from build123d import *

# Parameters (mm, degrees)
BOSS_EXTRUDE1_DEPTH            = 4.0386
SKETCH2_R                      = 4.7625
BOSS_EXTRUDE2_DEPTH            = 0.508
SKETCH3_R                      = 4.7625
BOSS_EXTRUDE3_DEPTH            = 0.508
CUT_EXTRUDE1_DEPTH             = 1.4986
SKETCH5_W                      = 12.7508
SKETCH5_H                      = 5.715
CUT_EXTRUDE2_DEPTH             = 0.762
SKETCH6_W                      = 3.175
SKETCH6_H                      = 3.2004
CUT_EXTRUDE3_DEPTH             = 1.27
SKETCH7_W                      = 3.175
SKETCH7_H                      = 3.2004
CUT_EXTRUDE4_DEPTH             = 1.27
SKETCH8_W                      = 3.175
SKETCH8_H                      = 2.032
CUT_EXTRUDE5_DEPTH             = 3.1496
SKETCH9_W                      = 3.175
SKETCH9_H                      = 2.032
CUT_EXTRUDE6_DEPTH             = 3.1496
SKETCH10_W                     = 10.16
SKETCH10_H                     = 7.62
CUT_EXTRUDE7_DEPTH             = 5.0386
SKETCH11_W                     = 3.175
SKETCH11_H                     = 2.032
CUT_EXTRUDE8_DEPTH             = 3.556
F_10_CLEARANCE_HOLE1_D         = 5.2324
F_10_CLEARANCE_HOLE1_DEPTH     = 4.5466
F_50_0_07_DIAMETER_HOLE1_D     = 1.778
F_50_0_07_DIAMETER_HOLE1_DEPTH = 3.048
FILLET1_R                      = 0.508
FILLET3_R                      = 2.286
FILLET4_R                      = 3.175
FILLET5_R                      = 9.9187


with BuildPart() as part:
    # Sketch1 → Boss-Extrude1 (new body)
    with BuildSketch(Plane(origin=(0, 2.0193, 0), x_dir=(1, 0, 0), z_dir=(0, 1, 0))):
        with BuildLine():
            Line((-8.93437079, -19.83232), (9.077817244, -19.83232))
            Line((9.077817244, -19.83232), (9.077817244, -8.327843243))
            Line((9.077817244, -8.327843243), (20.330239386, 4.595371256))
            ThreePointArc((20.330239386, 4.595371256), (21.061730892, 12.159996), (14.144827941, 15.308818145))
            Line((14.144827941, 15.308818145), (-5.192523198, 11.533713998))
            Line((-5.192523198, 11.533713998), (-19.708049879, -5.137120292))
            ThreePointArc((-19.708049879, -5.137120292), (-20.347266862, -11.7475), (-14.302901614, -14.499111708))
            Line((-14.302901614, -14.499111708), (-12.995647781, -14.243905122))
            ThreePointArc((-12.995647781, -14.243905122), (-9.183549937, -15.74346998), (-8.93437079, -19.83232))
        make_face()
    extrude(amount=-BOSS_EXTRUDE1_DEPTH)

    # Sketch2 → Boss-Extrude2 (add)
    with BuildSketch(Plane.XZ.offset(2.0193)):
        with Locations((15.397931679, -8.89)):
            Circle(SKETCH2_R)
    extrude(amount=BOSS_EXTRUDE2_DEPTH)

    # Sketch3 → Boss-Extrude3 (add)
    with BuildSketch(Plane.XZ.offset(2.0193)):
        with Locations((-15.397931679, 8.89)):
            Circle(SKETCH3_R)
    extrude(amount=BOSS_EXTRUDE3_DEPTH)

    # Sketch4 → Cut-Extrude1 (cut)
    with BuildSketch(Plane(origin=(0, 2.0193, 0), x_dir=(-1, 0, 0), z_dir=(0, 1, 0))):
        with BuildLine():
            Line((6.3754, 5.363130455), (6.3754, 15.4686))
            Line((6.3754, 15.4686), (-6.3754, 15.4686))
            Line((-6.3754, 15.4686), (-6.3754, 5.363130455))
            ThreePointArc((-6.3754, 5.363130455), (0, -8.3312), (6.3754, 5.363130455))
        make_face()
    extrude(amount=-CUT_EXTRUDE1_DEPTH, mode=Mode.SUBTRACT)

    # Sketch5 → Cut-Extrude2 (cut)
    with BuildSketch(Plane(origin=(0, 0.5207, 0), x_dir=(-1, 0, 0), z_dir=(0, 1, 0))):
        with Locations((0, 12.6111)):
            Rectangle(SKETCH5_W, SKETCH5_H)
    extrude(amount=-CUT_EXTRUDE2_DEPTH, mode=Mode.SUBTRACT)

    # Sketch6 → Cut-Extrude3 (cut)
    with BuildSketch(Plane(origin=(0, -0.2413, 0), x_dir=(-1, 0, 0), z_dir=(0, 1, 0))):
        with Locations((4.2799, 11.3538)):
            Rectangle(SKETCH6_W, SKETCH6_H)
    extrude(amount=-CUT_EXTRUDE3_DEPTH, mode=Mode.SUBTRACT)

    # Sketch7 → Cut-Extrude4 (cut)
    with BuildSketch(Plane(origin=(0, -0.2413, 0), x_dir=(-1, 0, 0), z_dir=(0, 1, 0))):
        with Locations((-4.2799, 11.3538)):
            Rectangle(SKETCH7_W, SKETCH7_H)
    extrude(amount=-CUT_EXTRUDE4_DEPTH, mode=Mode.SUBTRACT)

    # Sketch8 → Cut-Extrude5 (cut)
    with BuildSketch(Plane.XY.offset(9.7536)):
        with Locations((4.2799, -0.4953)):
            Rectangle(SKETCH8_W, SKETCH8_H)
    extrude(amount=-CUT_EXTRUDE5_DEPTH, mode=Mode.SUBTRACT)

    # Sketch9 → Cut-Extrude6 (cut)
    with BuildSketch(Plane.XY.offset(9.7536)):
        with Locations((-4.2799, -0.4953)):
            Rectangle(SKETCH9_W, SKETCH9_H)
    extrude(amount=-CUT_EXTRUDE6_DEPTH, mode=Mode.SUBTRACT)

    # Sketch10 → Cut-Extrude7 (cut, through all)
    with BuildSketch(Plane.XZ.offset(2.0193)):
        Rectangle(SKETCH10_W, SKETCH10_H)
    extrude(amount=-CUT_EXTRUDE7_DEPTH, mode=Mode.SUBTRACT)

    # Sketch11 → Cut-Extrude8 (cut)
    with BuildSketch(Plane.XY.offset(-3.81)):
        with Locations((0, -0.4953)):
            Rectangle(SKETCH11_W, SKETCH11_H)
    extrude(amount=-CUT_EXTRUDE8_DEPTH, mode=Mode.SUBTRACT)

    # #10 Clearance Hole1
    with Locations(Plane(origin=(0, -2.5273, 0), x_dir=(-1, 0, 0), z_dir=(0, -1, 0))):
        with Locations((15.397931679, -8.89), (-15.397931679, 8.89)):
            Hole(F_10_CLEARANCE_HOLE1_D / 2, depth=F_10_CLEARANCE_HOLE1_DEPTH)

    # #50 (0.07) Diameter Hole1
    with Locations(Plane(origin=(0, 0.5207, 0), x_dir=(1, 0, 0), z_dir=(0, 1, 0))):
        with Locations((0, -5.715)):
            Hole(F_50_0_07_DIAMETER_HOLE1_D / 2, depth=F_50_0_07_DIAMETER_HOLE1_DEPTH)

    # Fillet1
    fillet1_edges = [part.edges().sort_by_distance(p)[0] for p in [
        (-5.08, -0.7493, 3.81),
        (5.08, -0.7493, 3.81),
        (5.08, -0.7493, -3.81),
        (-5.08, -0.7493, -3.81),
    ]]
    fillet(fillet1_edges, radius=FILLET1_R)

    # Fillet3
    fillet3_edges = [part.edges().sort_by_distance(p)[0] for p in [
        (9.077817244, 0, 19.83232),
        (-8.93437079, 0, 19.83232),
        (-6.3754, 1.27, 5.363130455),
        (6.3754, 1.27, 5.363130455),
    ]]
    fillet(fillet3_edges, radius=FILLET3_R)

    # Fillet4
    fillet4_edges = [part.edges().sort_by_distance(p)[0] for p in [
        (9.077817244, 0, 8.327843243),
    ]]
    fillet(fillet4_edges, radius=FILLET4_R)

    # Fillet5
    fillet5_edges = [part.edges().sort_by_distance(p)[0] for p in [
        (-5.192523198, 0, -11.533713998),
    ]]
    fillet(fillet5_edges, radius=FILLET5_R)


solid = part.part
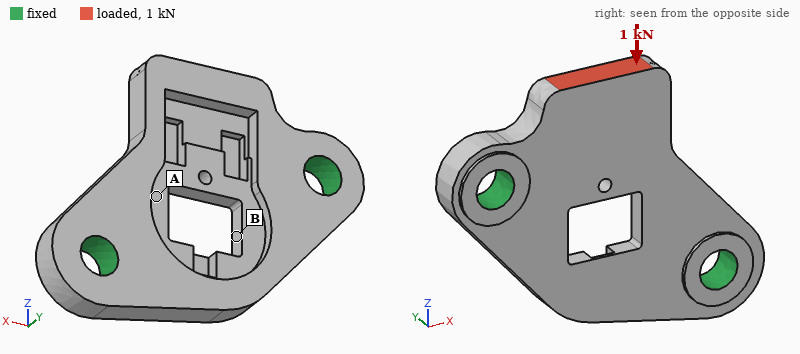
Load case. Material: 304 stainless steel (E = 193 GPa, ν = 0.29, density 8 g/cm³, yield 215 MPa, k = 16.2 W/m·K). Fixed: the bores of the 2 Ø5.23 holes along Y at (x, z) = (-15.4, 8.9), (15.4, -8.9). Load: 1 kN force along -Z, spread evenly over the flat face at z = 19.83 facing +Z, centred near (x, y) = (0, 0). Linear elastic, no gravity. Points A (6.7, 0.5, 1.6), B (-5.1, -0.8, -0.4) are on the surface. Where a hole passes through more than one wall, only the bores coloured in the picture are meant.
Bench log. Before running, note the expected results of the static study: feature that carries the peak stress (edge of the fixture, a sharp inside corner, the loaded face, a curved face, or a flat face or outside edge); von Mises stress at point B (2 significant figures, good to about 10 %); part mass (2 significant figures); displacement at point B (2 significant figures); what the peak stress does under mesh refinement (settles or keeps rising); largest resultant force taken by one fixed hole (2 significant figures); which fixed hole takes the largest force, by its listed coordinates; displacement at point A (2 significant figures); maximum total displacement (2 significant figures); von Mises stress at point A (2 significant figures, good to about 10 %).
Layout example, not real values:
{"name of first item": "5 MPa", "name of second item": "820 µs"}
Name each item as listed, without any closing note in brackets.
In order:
{"feature that carries the peak stress": "a sharp inside corner", "von Mises stress at point B": "9.4 MPa", "part mass": "23 g", "displacement at point B": "1.1 µm", "what the peak stress does under mesh refinement": "keeps rising", "largest resultant force taken by one fixed hole": "540 N", "which fixed hole takes the largest force, by its listed coordinates": "(15.4, -8.9)", "displacement at point A": "1.4 µm", "maximum total displacement": "7.3 µm", "von Mises stress at point A": "25 MPa"}
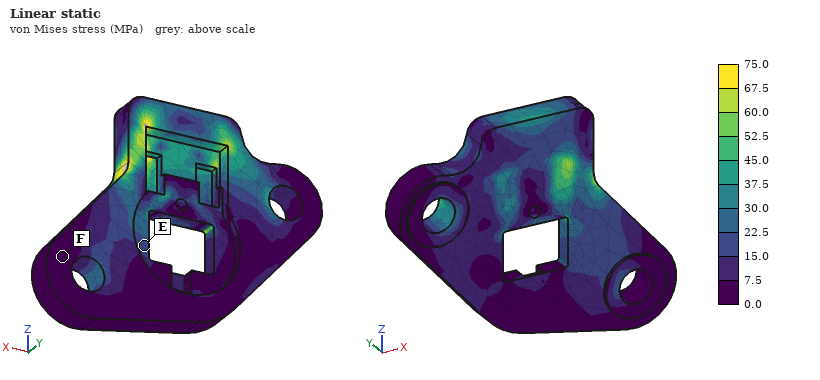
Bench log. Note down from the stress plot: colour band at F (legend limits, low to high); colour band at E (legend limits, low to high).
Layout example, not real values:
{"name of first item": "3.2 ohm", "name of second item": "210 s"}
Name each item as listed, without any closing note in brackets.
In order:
{"colour band at F": "0.0 to 7.5 MPa", "colour band at E": "15.0 to 22.5 MPa"}
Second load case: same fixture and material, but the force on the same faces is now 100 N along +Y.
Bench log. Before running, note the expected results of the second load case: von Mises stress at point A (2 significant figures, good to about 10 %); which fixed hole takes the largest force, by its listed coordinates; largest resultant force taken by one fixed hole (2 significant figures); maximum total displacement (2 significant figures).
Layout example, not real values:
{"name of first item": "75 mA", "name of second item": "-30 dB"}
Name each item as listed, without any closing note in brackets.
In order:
{"von Mises stress at point A": "11 MPa", "which fixed hole takes the largest force, by its listed coordinates": "(-15.4, 8.9)", "largest resultant force taken by one fixed hole": "89 N", "maximum total displacement": "18 µm"}
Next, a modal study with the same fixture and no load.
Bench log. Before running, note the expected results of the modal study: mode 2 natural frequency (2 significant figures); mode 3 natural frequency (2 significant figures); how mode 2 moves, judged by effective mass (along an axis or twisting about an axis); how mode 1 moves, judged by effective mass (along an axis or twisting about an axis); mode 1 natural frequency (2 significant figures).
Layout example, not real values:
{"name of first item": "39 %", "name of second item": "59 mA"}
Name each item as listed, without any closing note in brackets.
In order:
{"mode 2 natural frequency": "16 kHz", "mode 3 natural frequency": "21 kHz", "how mode 2 moves, judged by effective mass": "along Y", "how mode 1 moves, judged by effective mass": "along Y", "mode 1 natural frequency": "8100 Hz"}
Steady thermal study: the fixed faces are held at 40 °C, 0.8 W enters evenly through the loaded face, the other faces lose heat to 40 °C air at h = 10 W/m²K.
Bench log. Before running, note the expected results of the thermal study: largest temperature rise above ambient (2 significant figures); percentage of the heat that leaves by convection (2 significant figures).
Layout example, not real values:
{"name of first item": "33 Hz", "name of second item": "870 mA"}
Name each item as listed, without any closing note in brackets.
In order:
{"largest temperature rise above ambient": "18 K", "percentage of the heat that leaves by convection": "12 %"}
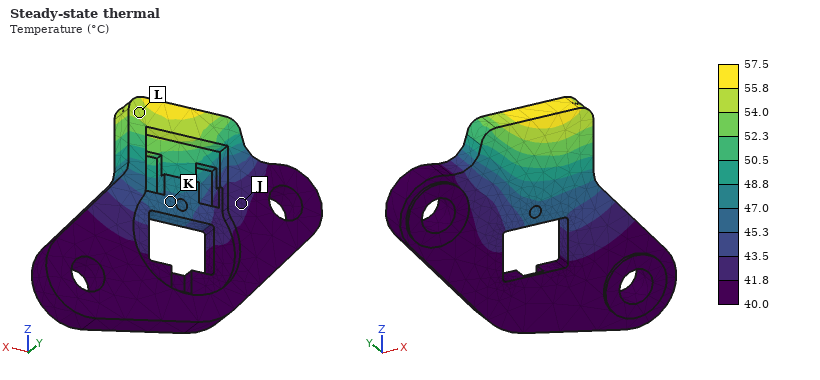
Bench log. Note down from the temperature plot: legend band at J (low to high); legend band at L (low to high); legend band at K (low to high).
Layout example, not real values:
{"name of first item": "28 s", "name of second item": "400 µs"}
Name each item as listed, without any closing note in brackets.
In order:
{"legend band at J": "41.8 to 43.5 °C", "legend band at L": "54.0 to 55.8 °C", "legend band at K": "45.3 to 47.0 °C"}
